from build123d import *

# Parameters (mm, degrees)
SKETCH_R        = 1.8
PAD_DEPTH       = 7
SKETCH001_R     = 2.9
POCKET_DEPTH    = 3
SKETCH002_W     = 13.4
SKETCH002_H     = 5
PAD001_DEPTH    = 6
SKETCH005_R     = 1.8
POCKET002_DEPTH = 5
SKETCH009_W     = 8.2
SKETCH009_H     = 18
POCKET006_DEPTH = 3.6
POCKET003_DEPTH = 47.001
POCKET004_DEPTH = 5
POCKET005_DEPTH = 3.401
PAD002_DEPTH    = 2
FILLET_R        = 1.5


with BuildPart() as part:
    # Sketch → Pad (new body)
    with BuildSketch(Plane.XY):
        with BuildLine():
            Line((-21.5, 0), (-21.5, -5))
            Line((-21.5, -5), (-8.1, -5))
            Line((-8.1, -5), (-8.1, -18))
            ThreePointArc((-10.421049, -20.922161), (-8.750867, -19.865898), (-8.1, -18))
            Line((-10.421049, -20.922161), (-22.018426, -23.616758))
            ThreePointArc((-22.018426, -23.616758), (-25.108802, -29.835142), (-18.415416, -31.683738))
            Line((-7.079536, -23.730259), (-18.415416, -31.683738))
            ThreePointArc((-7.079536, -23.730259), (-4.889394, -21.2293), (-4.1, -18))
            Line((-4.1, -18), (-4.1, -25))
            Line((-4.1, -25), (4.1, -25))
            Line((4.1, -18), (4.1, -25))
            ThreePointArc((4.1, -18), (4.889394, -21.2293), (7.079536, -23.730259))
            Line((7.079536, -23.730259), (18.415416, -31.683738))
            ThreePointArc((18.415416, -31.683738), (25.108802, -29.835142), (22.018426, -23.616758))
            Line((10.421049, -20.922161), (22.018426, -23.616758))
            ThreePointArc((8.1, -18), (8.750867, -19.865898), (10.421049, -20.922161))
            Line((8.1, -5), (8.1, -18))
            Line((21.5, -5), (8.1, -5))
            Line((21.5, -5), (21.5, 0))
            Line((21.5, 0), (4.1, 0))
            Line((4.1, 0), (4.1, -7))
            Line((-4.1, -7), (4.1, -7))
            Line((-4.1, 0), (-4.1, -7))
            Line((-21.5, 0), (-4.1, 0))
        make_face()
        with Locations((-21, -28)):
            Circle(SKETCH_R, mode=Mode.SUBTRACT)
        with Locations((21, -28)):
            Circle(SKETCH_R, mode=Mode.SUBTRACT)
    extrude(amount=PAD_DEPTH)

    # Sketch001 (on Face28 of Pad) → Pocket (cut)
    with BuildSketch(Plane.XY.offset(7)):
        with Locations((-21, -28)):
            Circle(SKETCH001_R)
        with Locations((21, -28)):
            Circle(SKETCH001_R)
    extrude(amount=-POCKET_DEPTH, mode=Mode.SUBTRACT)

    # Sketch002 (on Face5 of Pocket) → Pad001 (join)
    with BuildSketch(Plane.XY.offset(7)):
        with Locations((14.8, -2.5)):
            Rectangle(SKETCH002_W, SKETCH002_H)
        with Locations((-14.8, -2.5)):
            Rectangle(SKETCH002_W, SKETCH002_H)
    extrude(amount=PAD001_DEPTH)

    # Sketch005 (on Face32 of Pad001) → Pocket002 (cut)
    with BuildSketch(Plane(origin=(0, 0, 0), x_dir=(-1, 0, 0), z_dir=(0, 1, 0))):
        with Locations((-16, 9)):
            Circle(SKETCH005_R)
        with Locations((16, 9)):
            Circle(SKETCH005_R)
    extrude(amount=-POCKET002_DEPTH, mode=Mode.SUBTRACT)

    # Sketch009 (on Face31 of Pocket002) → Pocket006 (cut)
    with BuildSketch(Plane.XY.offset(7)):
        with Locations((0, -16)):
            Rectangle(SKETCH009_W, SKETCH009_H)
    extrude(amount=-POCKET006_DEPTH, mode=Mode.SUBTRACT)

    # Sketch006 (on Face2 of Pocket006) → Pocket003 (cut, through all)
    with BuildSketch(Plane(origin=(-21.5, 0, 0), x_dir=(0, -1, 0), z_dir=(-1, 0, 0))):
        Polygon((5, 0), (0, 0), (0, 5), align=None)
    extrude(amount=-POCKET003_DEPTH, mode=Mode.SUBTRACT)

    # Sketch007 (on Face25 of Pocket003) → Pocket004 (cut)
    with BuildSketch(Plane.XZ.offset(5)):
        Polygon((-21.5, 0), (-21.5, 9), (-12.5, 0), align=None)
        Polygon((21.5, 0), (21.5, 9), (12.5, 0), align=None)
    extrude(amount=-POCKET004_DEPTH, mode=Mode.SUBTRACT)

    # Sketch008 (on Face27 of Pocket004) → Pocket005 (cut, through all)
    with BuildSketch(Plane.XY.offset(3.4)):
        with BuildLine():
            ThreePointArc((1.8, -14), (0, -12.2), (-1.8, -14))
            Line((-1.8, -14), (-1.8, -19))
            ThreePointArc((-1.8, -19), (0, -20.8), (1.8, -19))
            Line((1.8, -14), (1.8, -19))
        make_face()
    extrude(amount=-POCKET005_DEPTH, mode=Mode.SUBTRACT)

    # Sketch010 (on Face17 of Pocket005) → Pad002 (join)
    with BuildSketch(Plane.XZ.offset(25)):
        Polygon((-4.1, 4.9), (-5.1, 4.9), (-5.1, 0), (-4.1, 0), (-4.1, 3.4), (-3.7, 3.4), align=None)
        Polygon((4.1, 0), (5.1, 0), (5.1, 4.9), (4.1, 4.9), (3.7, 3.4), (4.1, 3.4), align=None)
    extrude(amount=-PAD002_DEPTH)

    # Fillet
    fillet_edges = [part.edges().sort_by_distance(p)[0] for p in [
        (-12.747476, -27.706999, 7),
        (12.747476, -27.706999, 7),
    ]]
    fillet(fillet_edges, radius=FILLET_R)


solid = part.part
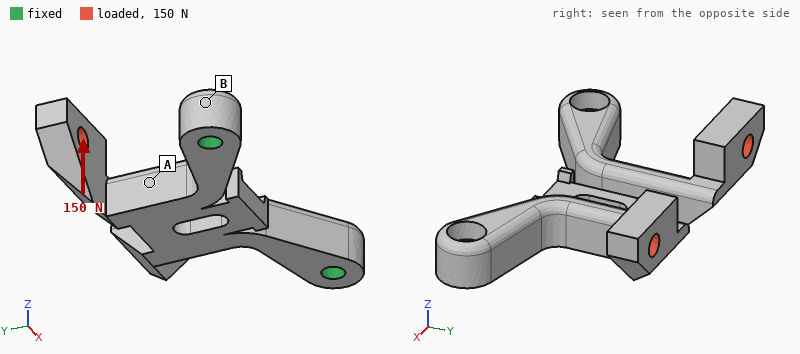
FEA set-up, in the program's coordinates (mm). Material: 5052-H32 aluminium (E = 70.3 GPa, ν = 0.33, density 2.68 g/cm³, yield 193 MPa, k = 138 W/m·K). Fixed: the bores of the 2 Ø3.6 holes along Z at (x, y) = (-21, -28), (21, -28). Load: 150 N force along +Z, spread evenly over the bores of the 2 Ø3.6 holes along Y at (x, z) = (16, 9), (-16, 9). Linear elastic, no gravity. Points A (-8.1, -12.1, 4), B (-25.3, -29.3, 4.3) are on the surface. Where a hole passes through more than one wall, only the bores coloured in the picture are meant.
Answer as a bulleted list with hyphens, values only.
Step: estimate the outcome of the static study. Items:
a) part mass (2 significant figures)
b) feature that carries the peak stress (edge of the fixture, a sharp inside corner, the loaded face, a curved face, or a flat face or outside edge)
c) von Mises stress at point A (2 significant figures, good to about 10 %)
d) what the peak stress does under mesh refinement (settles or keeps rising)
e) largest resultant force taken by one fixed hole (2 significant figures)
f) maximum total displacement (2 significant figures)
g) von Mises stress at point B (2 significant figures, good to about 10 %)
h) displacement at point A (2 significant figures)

- 11 g
- edge of the fixture
- 31 MPa
- keeps rising
- 77 N
- 0.21 mm
- 10 MPa
- 0.072 mm
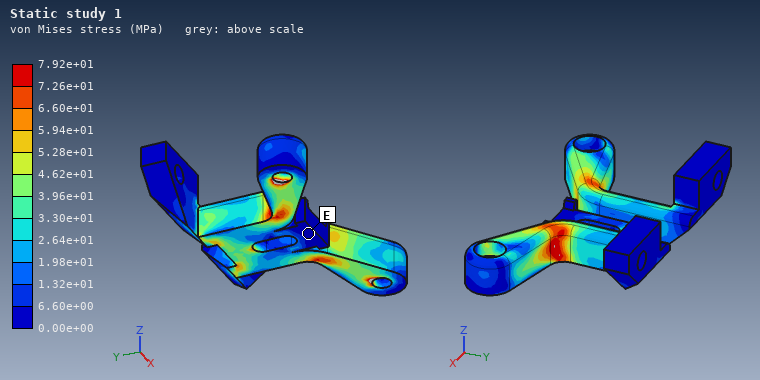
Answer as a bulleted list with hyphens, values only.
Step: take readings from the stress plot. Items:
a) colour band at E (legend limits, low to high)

- 0.00e+00 to 6.60e+00 MPa
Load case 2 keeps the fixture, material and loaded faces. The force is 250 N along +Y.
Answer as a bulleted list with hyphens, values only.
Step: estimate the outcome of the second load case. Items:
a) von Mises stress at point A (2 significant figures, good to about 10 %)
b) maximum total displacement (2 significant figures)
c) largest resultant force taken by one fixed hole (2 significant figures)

- 32 MPa
- 0.16 mm
- 130 N
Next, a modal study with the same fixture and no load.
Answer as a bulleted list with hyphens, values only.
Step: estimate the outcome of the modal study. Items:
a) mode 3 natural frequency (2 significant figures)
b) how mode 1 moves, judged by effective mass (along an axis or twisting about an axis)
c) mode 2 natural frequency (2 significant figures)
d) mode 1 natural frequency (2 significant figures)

- 4700 Hz
- along Z
- 3300 Hz
- 2500 Hz
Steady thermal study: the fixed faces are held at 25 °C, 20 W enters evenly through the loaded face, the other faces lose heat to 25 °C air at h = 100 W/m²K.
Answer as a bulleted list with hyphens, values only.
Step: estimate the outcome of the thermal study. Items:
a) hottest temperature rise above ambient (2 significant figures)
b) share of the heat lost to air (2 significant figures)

- 65 K
- 45 %
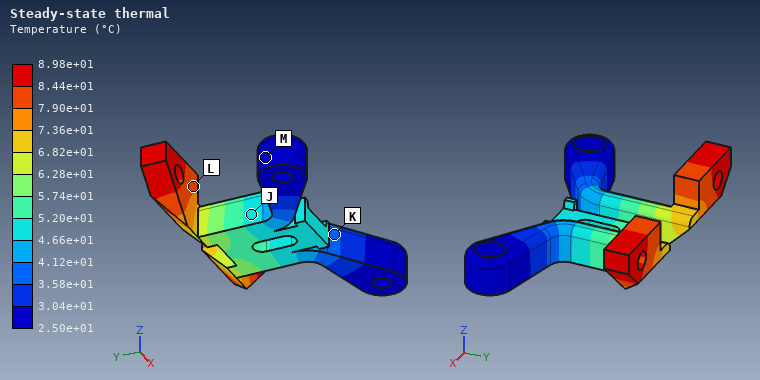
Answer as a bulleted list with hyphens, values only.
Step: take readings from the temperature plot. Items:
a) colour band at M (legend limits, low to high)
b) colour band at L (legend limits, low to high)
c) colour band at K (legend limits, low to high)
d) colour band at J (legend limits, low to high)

- 2.50e+01 to 3.04e+01 °C
- 7.90e+01 to 8.44e+01 °C
- 3.58e+01 to 4.12e+01 °C
- 4.66e+01 to 5.20e+01 °C
